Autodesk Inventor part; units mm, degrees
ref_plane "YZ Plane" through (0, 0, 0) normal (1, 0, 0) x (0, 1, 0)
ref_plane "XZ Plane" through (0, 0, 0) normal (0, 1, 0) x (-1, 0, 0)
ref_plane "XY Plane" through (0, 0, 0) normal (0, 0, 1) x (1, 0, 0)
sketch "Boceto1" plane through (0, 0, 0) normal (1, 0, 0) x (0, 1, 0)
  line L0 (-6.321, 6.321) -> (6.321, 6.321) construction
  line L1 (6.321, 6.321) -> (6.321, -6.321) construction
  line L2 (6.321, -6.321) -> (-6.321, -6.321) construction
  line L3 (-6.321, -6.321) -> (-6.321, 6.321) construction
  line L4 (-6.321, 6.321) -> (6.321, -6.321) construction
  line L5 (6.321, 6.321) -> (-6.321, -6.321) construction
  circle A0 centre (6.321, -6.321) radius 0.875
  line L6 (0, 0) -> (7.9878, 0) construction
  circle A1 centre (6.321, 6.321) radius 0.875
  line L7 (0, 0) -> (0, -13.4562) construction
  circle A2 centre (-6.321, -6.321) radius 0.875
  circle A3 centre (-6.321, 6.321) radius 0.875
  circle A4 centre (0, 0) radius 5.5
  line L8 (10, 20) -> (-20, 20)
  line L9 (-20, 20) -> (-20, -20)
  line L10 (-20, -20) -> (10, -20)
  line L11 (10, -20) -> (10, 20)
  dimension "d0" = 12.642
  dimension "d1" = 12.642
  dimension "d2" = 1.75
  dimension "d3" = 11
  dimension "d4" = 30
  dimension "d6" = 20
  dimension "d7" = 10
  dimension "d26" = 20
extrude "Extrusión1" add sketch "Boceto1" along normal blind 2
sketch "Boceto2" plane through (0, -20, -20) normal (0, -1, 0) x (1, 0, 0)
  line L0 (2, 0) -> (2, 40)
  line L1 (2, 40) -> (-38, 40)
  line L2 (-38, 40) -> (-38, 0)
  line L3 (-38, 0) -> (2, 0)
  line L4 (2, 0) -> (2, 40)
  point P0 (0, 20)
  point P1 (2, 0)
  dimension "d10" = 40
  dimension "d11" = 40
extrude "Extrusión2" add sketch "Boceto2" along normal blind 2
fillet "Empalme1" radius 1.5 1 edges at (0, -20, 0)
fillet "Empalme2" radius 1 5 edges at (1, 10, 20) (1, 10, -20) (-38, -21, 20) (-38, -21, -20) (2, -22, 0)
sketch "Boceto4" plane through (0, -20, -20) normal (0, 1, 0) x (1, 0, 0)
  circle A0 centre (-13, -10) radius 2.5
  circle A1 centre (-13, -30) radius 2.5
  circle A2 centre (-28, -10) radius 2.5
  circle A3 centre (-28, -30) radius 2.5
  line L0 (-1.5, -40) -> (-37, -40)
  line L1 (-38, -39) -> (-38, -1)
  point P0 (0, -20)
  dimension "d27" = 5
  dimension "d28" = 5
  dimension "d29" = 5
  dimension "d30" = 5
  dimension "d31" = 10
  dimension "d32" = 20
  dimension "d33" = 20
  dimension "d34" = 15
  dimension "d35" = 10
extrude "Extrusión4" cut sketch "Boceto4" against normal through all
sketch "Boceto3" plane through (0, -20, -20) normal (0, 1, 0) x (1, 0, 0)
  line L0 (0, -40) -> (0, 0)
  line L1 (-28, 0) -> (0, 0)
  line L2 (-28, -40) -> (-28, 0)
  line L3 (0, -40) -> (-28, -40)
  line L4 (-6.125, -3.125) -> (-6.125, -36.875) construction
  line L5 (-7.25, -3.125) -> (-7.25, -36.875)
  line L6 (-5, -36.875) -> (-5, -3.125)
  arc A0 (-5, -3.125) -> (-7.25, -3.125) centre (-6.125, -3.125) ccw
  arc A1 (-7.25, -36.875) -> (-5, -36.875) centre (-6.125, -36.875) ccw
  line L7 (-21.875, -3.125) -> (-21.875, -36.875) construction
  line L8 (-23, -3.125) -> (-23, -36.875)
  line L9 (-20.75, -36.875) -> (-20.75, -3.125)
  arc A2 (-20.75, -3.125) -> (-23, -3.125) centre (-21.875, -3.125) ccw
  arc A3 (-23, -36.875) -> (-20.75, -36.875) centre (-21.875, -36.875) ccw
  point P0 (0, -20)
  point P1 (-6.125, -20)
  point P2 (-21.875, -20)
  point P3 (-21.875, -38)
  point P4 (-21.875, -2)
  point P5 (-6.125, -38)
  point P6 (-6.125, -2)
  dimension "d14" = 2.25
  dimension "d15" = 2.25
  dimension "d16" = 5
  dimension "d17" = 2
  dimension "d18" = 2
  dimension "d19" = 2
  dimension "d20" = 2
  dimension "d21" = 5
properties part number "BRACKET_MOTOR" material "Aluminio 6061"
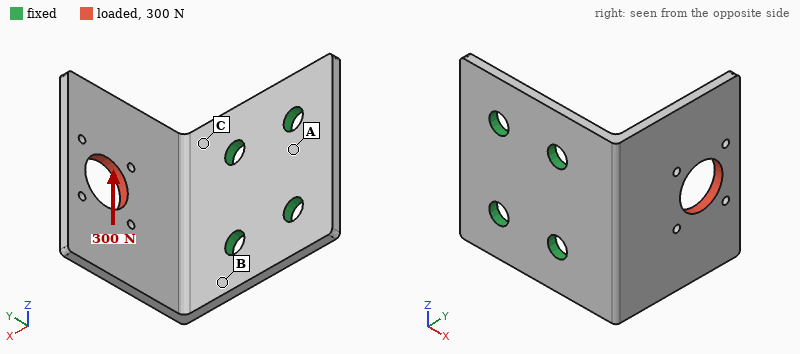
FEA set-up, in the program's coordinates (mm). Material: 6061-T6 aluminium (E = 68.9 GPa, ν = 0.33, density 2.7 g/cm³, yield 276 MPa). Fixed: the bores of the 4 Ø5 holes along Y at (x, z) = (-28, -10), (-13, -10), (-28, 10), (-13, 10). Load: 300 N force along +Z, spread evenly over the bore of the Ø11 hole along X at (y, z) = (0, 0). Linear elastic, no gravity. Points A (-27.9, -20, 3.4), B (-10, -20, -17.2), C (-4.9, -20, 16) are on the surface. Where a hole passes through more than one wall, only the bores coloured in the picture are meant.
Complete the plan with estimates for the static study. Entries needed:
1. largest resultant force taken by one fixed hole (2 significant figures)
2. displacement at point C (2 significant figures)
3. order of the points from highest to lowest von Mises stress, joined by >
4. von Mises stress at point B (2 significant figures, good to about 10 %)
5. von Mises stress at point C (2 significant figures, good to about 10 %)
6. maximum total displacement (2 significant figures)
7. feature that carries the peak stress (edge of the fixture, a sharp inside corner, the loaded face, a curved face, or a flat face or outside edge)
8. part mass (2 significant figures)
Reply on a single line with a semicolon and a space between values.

340 N; 0.065 mm; B > C > A; 88 MPa; 46 MPa; 0.33 mm; a flat face or outside edge; 14 g
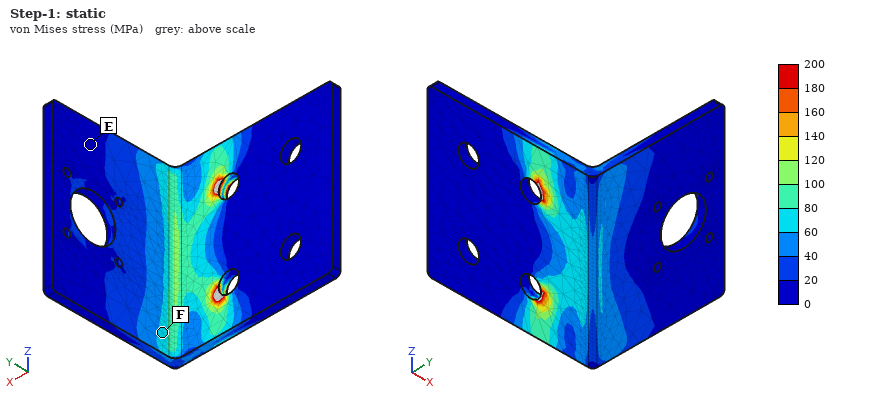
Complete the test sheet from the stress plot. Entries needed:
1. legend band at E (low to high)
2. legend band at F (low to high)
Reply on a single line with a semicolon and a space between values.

0 to 20 MPa; 60 to 80 MPa
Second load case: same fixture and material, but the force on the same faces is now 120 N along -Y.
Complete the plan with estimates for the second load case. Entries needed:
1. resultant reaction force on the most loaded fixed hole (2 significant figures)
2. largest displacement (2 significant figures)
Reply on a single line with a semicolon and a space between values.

67 N; 0.16 mm
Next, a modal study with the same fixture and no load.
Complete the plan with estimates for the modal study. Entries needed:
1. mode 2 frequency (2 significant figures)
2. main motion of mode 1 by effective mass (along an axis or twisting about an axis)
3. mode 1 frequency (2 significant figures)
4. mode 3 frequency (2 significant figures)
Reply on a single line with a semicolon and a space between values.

2300 Hz; along X; 1200 Hz; 3500 Hz
